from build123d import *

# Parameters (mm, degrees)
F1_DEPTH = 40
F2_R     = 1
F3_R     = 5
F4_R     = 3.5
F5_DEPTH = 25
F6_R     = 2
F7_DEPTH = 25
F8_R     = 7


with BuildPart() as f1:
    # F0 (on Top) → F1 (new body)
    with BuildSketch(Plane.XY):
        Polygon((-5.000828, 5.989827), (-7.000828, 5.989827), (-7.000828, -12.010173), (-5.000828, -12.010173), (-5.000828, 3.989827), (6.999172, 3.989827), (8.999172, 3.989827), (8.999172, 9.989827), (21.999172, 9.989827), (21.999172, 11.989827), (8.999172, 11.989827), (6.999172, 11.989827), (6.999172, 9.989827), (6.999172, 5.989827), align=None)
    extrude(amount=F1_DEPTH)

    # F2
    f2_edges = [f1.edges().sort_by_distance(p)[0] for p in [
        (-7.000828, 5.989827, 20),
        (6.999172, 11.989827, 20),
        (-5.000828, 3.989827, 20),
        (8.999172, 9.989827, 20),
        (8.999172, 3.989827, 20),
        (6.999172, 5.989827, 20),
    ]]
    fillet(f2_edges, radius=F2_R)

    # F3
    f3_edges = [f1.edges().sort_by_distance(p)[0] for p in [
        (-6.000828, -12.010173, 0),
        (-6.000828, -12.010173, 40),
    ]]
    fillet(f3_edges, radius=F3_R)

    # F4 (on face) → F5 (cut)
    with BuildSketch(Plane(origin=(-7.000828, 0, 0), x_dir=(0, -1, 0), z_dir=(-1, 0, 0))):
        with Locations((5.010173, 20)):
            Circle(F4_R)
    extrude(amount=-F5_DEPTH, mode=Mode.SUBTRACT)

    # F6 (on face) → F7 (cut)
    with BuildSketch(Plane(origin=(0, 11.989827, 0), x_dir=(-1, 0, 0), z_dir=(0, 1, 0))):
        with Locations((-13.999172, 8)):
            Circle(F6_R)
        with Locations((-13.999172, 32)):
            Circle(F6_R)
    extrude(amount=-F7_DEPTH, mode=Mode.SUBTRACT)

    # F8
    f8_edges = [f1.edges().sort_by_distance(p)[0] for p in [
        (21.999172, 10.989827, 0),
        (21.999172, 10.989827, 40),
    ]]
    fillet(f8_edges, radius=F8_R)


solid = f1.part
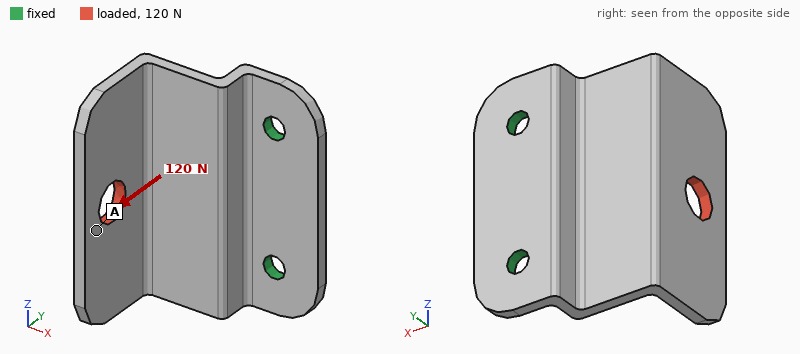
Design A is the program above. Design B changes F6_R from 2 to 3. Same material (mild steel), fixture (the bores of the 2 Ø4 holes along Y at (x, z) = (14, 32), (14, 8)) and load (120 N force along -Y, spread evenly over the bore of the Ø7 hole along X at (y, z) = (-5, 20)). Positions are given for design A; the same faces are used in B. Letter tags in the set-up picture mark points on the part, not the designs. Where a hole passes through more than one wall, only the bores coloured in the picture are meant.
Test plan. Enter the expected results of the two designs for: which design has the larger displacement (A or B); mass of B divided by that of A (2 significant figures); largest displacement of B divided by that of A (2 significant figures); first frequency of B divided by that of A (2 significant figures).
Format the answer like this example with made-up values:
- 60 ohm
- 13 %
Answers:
- A
- 0.98
- 0.87
- 1.1
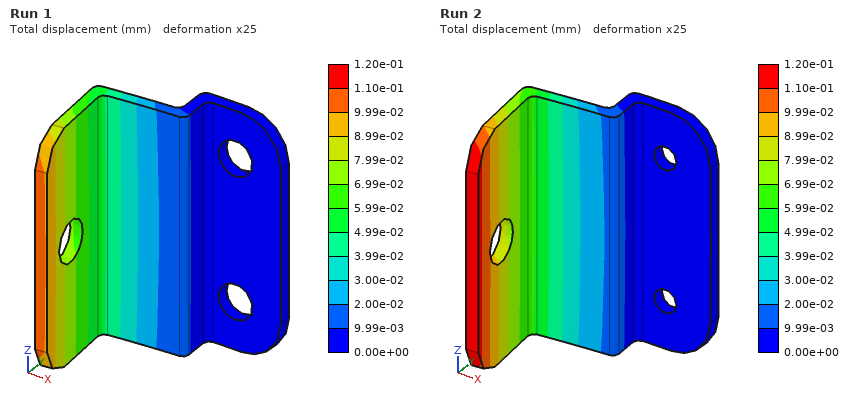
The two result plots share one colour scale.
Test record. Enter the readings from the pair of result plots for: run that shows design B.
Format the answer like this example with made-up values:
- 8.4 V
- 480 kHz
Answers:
- Run 1
